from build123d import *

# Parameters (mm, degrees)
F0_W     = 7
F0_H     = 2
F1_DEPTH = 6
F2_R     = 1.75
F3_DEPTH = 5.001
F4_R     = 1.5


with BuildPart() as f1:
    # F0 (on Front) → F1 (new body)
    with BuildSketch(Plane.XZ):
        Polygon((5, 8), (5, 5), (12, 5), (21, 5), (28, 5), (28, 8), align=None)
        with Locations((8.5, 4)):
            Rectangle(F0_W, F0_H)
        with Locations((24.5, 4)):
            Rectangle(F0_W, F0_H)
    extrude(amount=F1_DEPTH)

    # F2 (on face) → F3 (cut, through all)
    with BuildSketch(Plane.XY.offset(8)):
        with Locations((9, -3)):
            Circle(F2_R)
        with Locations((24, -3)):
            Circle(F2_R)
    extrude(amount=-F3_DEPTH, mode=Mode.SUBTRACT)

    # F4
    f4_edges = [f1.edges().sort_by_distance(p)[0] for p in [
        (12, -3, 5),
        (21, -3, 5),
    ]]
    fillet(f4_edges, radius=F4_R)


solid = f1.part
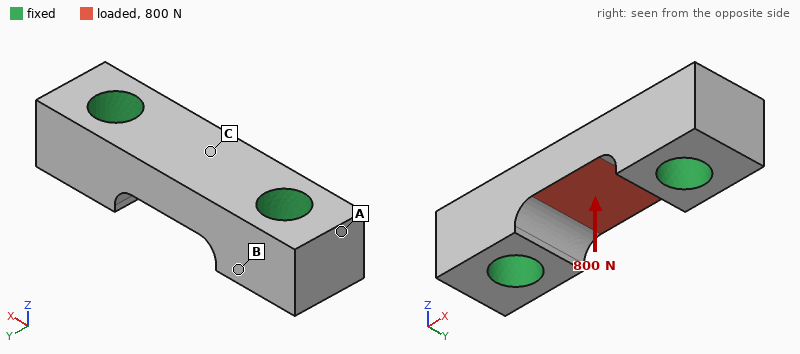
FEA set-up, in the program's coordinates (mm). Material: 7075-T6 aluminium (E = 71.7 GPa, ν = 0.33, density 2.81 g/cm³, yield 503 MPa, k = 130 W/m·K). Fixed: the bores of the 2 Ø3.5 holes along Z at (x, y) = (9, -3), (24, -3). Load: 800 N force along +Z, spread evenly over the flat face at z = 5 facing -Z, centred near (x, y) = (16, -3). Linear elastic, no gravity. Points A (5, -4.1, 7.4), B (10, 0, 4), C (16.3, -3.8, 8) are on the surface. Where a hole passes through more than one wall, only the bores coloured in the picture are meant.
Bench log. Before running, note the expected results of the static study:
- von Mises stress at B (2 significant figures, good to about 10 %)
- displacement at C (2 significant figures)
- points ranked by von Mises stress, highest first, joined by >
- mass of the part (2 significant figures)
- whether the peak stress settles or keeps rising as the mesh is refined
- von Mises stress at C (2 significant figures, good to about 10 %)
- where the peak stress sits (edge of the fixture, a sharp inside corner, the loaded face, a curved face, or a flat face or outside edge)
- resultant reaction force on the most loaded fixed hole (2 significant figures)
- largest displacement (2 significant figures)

18 MPa
6.7 µm
C > B > A
1.4 g
keeps rising
64 MPa
edge of the fixture
410 N
7.9 µm
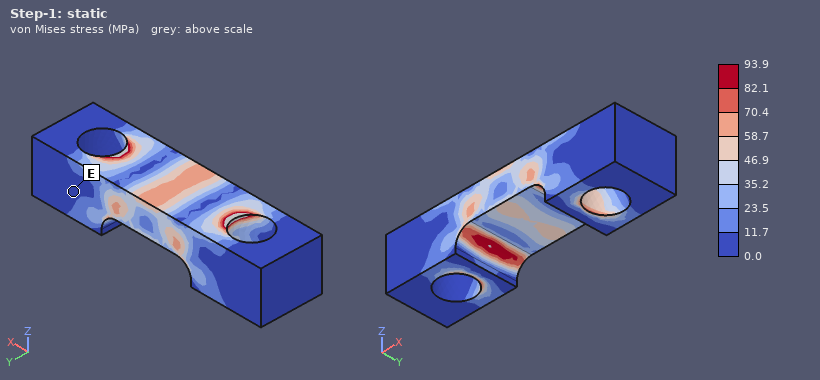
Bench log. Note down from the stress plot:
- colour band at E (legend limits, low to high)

0.0 to 11.7 MPa
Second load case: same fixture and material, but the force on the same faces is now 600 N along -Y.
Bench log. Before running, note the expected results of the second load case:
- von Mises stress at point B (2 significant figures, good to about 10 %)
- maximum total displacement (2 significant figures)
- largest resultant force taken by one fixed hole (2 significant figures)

15 MPa
8.2 µm
300 N
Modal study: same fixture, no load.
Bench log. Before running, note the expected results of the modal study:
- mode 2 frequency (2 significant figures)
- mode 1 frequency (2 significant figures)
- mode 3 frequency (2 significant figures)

99 kHz
97 kHz
120 kHz
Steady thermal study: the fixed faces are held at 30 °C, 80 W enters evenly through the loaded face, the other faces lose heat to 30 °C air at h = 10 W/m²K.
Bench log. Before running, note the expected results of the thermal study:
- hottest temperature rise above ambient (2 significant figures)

88 K
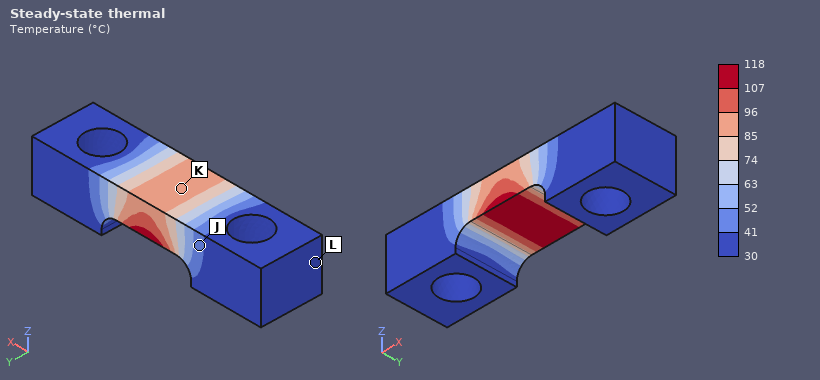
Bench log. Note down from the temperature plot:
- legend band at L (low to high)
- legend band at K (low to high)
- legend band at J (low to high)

30 to 41 °C
85 to 96 °C
41 to 52 °C
